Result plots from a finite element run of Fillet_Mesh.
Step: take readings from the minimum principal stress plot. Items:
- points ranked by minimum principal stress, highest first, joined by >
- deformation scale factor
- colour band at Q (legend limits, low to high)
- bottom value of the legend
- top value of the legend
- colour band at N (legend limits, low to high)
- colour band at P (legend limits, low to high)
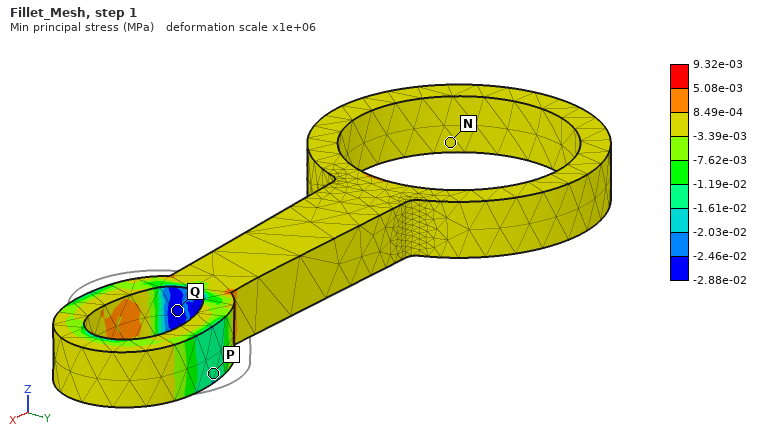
N > P > Q
1e+06
-2.88e-02 to -2.46e-02 MPa
-2.88e-02 MPa
9.32e-03 MPa
-3.39e-03 to 8.49e-04 MPa
-1.61e-02 to -1.19e-02 MPa
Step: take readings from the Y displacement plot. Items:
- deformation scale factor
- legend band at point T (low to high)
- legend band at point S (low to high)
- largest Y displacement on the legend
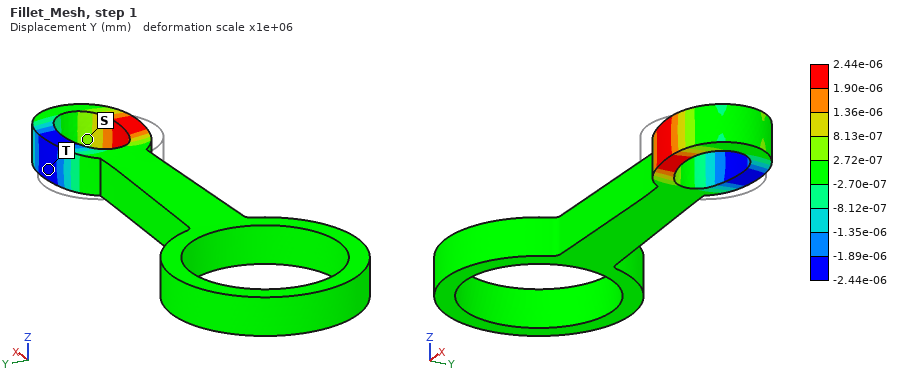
1e+06
-2.44e-06 to -1.89e-06 mm
2.72e-07 to 8.13e-07 mm
2.44e-06 mm
